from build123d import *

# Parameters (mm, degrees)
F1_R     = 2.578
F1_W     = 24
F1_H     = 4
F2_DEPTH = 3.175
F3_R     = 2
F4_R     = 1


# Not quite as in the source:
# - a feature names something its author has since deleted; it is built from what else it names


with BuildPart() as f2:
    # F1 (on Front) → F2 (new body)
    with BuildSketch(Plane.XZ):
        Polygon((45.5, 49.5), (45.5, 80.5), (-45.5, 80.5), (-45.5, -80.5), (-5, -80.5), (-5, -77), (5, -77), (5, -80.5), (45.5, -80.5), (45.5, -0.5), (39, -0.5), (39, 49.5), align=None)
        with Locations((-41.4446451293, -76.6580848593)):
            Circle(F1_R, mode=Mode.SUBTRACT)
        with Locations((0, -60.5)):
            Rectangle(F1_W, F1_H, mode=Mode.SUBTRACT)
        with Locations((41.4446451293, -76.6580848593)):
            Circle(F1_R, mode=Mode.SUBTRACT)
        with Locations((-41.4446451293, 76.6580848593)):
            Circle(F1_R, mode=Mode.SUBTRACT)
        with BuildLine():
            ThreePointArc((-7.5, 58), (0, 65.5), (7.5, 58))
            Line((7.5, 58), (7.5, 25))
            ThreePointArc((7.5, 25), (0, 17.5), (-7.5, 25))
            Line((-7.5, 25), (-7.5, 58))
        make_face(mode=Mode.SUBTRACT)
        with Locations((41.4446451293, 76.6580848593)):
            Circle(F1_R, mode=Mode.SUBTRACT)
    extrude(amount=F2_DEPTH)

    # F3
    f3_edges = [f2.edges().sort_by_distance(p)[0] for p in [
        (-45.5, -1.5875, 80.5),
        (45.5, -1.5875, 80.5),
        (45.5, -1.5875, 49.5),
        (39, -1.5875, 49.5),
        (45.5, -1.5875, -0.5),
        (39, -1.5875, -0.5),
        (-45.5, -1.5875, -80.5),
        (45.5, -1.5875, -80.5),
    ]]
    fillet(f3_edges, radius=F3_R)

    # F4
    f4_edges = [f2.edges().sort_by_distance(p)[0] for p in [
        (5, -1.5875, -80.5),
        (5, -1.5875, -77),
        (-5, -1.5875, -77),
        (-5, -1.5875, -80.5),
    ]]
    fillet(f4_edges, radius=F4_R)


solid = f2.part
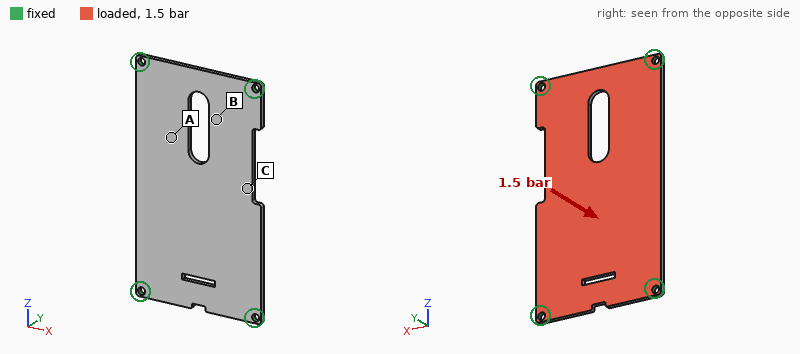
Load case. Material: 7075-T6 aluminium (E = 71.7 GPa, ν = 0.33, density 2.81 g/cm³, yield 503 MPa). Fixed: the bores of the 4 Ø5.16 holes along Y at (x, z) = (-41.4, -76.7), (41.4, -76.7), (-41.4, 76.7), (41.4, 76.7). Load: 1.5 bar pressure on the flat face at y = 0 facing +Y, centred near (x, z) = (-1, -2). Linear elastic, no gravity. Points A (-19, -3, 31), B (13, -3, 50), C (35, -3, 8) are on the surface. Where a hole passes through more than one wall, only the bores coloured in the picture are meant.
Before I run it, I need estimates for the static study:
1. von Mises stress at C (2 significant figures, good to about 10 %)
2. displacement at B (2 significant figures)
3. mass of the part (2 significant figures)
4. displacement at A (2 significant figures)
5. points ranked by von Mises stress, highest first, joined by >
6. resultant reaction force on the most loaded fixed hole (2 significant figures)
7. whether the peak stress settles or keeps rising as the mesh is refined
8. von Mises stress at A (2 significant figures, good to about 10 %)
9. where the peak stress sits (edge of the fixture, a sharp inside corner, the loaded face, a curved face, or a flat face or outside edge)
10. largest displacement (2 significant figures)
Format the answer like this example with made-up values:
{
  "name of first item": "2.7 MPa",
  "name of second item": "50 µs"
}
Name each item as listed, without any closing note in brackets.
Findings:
{
  "von Mises stress at C": "130 MPa",
  "displacement at B": "0.86 mm",
  "mass of the part": "120 g",
  "displacement at A": "1.3 mm",
  "points ranked by von Mises stress, highest first, joined by >": "C > A > B",
  "resultant reaction force on the most loaded fixed hole": "520 N",
  "whether the peak stress settles or keeps rising as the mesh is refined": "keeps rising",
  "von Mises stress at A": "73 MPa",
  "where the peak stress sits": "edge of the fixture",
  "largest displacement": "1.7 mm"
}
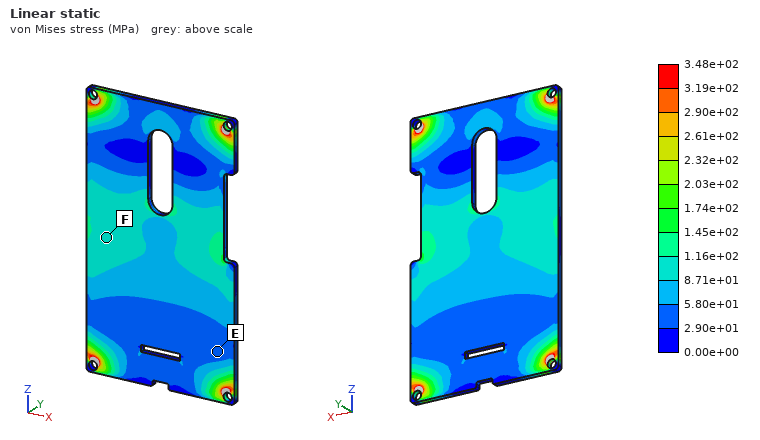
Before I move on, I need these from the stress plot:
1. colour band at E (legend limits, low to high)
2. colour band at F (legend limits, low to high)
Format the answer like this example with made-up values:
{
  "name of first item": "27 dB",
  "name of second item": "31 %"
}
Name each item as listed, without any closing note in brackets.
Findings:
{
  "colour band at E": "2.90e+01 to 5.80e+01 MPa",
  "colour band at F": "8.71e+01 to 1.16e+02 MPa"
}
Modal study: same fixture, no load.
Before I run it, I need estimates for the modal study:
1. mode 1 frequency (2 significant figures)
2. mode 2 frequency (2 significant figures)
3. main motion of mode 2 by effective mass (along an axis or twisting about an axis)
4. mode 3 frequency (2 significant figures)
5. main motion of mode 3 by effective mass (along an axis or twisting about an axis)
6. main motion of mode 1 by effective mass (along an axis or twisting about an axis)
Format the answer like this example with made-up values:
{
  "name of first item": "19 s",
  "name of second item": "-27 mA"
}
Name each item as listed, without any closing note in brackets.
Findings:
{
  "mode 1 frequency": "570 Hz",
  "mode 2 frequency": "1000 Hz",
  "main motion of mode 2 by effective mass": "twisting about Z",
  "mode 3 frequency": "1500 Hz",
  "main motion of mode 3 by effective mass": "twisting about X",
  "main motion of mode 1 by effective mass": "along Y"
}
